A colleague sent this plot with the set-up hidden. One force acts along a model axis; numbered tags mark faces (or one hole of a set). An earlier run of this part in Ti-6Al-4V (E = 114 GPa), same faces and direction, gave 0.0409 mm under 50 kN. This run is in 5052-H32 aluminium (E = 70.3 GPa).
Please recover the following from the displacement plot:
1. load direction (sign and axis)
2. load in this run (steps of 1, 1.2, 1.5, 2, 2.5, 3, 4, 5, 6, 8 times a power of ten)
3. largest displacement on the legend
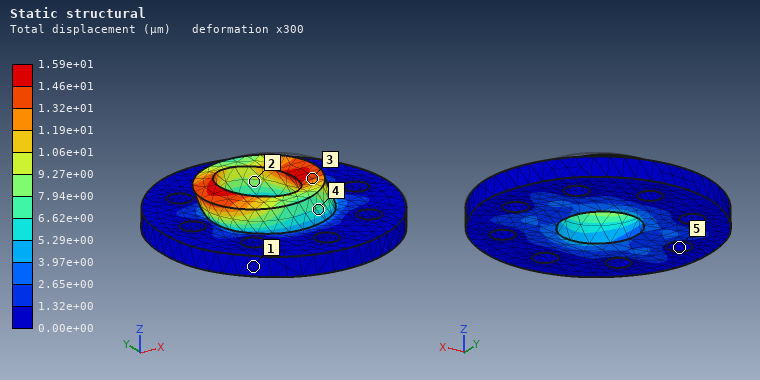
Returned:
-X
12 kN
1.59e+01 µm
